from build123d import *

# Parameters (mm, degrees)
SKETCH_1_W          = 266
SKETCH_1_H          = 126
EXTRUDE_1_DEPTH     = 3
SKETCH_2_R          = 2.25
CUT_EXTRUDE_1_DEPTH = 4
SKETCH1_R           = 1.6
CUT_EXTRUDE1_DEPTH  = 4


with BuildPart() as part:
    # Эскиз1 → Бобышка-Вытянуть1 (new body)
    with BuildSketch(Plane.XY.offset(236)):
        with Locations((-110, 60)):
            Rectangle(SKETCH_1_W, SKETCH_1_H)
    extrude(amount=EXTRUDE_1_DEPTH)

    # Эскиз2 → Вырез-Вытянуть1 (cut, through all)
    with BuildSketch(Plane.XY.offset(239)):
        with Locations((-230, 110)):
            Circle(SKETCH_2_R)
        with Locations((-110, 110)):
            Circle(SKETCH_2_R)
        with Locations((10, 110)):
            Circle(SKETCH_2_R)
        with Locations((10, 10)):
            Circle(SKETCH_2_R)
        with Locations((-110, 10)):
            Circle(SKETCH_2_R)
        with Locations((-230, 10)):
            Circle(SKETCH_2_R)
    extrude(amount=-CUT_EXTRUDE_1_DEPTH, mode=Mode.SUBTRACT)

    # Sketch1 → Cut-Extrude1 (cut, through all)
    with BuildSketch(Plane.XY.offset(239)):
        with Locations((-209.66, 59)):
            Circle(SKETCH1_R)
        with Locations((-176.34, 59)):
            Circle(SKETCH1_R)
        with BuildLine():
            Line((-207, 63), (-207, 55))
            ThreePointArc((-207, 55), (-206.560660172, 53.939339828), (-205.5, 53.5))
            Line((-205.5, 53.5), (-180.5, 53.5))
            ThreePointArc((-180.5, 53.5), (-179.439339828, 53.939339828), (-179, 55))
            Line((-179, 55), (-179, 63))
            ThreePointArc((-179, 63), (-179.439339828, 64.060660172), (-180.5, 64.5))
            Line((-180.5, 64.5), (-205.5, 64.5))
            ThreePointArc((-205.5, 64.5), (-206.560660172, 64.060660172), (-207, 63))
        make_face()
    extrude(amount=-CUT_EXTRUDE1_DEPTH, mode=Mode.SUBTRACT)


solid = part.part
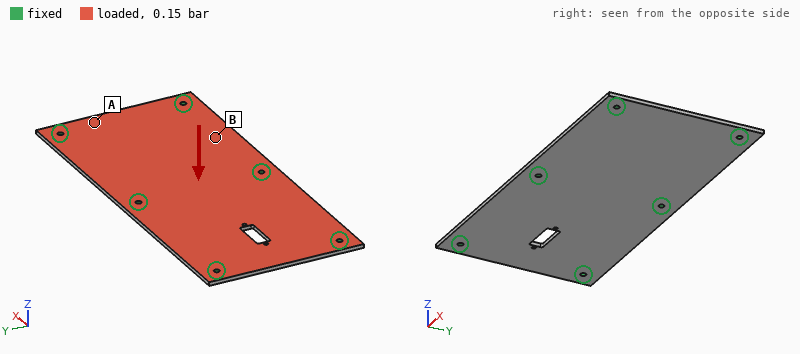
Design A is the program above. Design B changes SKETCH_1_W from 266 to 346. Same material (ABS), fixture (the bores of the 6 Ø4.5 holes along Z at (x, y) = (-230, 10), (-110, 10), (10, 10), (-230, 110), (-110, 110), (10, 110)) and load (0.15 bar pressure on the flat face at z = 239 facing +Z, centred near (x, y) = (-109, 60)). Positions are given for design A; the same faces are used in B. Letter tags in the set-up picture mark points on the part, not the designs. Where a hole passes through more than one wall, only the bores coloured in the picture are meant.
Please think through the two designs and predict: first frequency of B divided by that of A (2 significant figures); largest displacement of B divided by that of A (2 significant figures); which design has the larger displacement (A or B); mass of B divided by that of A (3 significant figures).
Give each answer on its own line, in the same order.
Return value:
0.80
1.5
B
1.30
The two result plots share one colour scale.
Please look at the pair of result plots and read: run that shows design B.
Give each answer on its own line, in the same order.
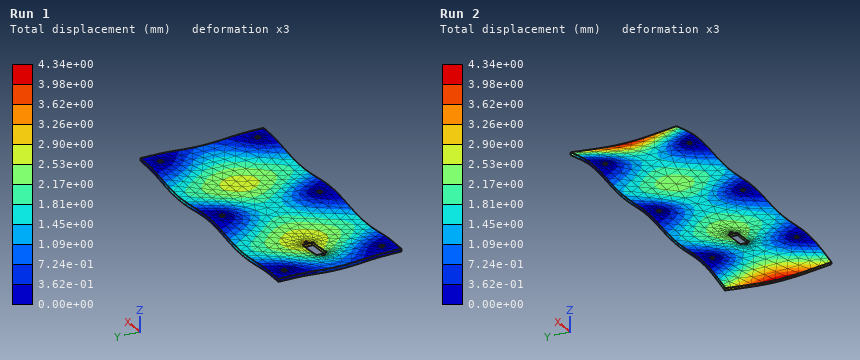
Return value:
Run 2
